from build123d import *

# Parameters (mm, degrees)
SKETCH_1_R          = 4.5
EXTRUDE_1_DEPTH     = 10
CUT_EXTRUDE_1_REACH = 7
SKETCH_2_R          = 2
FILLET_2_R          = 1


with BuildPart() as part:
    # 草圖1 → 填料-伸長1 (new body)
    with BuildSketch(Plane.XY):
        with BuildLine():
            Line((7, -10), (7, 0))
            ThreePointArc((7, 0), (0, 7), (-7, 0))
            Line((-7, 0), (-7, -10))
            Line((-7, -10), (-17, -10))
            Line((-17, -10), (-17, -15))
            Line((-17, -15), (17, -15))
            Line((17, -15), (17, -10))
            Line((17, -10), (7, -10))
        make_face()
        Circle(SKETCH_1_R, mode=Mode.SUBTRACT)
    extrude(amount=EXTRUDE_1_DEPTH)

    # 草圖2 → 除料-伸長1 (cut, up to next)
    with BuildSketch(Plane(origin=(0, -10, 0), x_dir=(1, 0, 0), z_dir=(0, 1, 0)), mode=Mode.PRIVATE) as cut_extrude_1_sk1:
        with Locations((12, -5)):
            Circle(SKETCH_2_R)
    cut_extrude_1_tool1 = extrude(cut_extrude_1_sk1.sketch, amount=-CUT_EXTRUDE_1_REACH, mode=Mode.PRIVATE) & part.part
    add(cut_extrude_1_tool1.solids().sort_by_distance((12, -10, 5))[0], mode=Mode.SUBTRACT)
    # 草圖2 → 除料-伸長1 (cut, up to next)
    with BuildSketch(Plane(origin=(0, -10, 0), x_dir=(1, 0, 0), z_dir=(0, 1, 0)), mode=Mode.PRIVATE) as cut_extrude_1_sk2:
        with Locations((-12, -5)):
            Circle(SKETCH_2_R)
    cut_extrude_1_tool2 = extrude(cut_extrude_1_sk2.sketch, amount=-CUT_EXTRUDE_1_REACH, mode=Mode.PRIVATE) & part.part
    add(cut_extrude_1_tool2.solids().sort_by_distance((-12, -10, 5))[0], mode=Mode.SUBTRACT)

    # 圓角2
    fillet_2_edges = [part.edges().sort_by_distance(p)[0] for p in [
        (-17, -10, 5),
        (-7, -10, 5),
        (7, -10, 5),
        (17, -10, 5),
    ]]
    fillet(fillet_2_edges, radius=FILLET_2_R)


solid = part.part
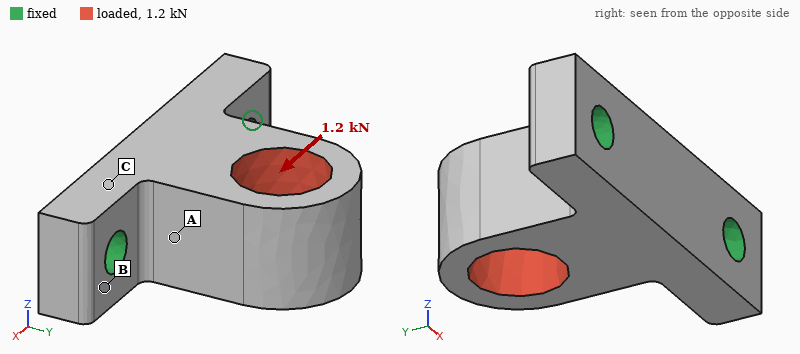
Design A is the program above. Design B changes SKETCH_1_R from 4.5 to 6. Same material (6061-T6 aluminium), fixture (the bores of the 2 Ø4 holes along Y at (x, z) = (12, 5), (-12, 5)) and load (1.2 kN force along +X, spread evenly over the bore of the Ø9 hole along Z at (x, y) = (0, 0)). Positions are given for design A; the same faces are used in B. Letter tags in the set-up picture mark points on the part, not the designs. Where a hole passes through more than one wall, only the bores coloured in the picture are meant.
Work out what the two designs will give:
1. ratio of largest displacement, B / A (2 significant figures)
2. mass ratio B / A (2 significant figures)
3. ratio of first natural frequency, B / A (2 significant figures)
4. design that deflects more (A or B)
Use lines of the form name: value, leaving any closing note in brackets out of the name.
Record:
ratio of largest displacement, B / A: 5.5
mass ratio B / A: 0.84
ratio of first natural frequency, B / A: 1.1
design that deflects more: B
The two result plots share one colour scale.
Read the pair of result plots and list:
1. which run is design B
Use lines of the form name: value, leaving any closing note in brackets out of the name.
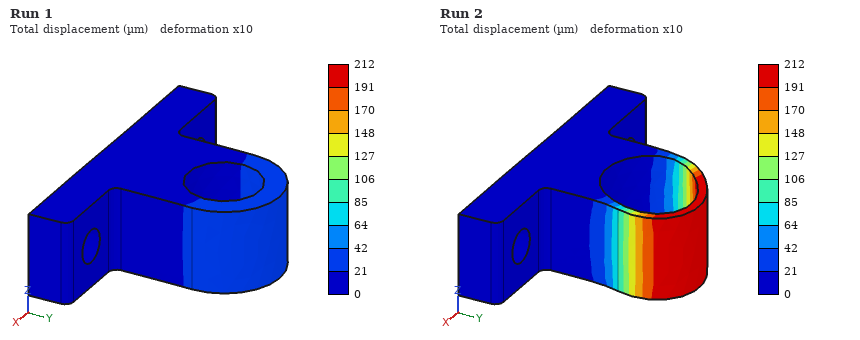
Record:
which run is design B: Run 2
